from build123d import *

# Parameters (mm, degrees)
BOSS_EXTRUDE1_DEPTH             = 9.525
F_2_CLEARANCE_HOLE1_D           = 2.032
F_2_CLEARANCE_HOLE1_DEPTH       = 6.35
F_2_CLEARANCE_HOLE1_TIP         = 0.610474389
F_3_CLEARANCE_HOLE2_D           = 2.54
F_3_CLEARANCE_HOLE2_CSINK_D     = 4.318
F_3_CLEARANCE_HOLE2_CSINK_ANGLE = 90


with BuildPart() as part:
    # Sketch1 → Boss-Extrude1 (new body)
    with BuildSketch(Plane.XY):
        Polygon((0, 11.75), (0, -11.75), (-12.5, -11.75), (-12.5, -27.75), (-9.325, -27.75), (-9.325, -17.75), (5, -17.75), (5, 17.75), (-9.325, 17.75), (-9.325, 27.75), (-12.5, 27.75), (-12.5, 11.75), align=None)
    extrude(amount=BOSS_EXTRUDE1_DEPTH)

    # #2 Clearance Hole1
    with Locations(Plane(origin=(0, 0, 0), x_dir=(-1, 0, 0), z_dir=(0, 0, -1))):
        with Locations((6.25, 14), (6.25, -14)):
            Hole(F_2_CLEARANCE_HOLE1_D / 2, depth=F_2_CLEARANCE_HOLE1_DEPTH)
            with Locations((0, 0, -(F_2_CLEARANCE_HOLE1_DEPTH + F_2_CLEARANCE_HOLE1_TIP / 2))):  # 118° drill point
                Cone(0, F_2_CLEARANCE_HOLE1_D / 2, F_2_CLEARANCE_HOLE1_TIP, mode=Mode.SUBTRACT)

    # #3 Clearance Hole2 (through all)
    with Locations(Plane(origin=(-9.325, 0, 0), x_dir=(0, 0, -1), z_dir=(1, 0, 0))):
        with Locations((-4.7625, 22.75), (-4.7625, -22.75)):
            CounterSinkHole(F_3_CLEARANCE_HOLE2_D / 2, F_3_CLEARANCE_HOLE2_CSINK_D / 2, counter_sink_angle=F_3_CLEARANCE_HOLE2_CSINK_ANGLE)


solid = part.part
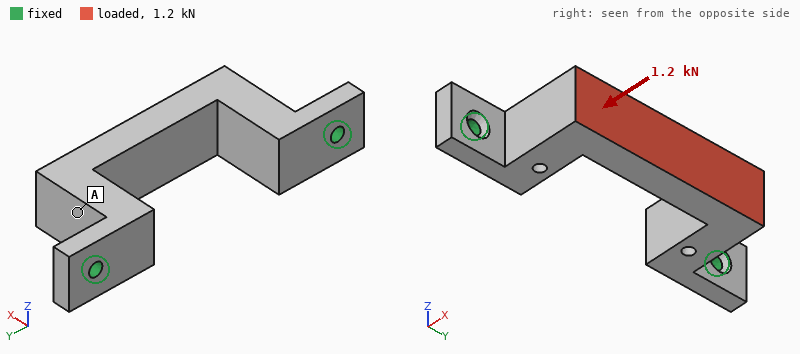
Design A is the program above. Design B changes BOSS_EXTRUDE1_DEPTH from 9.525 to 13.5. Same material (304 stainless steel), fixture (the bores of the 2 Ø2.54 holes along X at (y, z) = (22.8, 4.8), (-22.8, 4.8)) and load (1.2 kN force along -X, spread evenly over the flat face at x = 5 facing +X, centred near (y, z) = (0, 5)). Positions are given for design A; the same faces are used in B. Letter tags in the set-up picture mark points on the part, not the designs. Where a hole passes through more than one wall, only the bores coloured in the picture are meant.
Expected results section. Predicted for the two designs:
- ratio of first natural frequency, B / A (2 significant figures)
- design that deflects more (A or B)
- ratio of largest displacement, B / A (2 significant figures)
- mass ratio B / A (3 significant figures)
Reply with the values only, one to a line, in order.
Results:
0.92
B
1.8
1.43
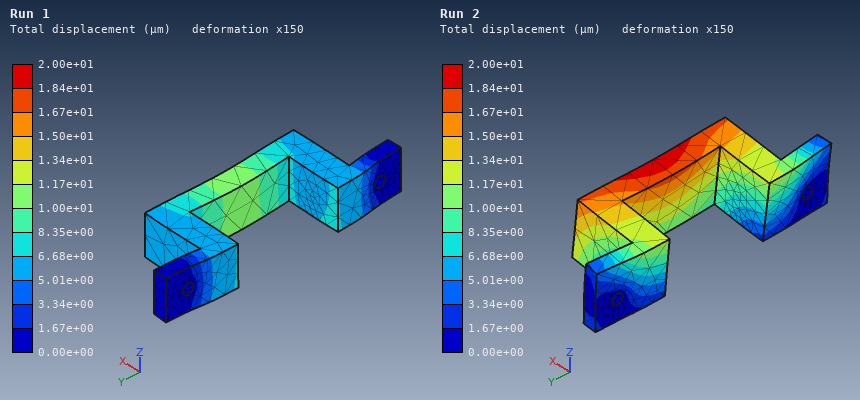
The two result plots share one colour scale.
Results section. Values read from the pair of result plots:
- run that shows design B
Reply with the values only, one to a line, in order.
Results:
Run 2
